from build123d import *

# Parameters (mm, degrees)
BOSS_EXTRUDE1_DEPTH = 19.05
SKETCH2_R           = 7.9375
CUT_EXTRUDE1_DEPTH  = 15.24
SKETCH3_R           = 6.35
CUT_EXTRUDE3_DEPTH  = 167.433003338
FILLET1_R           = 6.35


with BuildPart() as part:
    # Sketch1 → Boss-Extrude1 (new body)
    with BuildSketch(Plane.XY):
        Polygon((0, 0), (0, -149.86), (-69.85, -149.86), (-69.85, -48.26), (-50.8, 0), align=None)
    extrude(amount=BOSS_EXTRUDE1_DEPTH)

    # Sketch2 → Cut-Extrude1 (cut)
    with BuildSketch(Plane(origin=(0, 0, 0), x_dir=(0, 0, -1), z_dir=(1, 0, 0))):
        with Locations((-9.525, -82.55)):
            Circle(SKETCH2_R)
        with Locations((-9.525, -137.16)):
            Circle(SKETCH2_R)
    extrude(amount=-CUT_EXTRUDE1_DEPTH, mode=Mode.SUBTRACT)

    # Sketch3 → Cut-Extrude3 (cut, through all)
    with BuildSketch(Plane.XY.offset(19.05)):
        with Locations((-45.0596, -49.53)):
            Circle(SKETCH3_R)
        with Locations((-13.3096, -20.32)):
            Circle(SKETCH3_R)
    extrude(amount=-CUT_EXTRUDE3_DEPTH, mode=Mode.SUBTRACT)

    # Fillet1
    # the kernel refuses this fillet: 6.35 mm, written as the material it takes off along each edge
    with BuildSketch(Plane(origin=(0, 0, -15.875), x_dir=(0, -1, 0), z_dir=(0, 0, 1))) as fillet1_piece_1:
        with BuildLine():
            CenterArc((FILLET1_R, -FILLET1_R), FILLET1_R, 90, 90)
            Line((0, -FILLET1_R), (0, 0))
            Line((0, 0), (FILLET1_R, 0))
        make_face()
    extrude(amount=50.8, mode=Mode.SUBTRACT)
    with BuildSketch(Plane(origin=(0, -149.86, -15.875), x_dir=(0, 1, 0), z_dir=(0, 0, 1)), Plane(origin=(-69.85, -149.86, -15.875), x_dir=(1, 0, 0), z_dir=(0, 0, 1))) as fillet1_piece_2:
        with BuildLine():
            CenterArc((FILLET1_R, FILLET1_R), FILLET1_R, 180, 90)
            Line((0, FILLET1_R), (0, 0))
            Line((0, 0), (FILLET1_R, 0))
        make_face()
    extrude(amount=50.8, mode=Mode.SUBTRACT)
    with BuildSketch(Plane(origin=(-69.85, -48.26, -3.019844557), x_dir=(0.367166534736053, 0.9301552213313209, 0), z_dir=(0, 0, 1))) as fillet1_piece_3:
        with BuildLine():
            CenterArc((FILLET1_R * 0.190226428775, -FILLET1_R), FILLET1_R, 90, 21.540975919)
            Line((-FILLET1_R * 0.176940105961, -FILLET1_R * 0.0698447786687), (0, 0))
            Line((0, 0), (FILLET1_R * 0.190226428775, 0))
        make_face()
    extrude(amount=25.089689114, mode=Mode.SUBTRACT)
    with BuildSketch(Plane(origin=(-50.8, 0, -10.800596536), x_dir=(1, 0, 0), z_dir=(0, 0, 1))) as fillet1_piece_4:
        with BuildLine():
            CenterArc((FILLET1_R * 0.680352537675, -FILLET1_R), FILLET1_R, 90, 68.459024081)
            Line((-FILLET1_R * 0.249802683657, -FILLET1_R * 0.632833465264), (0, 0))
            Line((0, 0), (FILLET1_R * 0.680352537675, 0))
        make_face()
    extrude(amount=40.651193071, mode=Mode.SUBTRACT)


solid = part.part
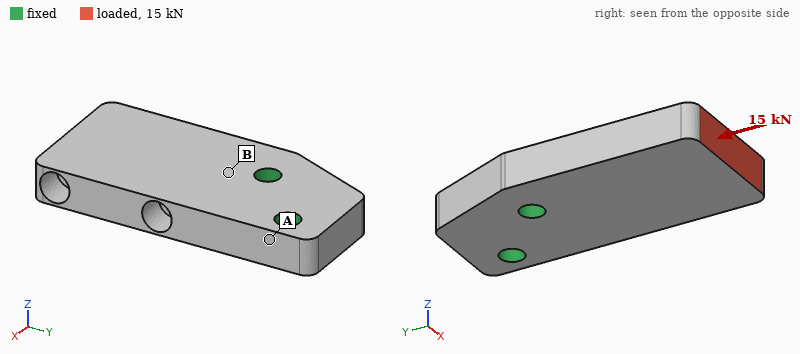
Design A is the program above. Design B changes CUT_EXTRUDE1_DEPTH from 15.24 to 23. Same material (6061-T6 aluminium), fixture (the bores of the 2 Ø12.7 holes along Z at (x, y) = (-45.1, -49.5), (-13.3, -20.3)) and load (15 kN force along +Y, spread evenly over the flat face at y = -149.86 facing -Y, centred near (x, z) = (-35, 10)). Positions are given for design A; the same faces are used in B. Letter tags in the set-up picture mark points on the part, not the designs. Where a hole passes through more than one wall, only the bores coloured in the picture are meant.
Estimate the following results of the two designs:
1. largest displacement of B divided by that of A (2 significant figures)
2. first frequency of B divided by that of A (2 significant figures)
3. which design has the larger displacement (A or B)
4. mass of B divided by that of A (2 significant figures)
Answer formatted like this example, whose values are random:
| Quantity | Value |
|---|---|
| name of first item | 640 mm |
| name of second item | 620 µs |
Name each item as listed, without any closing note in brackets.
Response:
| Quantity | Value |
|---|---|
| largest displacement of B divided by that of A | 1.3 |
| first frequency of B divided by that of A | 1.0 |
| which design has the larger displacement | B |
| mass of B divided by that of A | 0.98 |
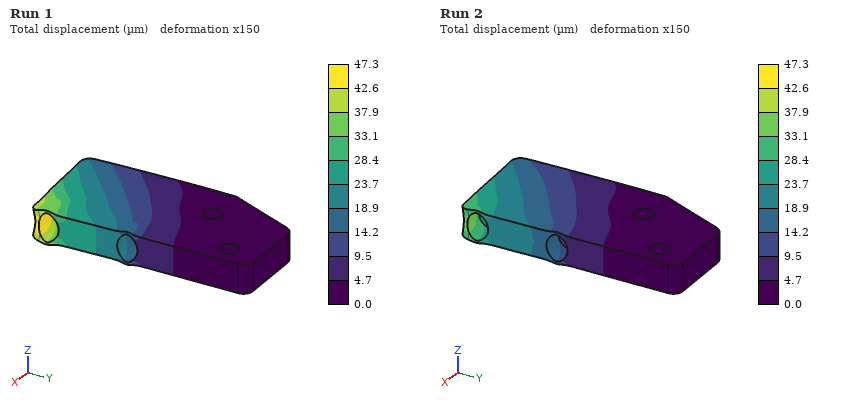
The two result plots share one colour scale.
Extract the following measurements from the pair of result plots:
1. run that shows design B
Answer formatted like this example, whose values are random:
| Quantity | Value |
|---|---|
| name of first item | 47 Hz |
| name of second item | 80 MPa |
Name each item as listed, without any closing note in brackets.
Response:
| Quantity | Value |
|---|---|
| run that shows design B | Run 1 |
